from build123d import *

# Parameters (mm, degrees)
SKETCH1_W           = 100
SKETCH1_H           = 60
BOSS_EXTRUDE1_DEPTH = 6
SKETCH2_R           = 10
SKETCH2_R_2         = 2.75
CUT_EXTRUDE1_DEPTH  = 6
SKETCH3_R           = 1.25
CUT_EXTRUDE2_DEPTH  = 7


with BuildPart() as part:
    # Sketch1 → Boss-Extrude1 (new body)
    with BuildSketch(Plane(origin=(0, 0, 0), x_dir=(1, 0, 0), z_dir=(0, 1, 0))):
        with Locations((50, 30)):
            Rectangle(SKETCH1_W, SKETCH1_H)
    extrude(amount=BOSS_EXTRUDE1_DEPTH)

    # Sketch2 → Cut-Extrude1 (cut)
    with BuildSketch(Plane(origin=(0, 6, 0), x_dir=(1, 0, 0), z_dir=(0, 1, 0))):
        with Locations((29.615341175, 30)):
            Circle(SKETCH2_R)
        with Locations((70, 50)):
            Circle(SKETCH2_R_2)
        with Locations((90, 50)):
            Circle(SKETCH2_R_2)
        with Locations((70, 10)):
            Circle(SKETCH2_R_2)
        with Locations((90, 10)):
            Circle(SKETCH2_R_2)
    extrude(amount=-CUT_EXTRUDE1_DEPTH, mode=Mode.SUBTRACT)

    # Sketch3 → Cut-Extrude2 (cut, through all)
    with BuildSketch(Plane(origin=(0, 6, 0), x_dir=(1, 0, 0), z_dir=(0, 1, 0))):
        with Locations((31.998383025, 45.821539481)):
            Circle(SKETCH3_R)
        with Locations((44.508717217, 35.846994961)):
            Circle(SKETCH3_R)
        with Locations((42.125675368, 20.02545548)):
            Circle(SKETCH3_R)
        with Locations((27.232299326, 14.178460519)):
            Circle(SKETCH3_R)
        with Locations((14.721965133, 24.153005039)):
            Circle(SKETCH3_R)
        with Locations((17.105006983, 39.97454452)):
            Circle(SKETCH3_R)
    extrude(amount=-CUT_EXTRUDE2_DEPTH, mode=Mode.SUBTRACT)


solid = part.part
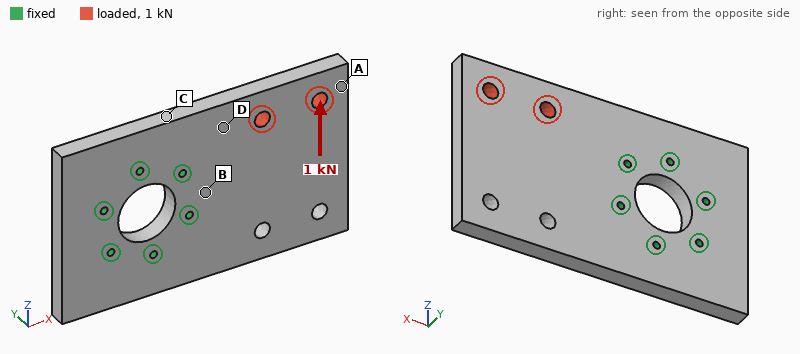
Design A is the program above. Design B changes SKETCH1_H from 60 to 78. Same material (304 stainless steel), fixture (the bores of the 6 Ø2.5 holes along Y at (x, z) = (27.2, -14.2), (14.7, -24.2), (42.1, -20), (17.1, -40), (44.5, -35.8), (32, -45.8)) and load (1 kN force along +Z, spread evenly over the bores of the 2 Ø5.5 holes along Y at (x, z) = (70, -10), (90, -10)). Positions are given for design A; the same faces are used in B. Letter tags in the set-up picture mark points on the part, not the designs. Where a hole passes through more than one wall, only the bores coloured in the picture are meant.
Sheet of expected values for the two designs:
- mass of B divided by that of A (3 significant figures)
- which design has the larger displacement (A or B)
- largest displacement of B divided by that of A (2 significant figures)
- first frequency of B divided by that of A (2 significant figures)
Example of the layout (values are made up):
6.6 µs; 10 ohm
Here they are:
1.32; A; 0.81; 0.95
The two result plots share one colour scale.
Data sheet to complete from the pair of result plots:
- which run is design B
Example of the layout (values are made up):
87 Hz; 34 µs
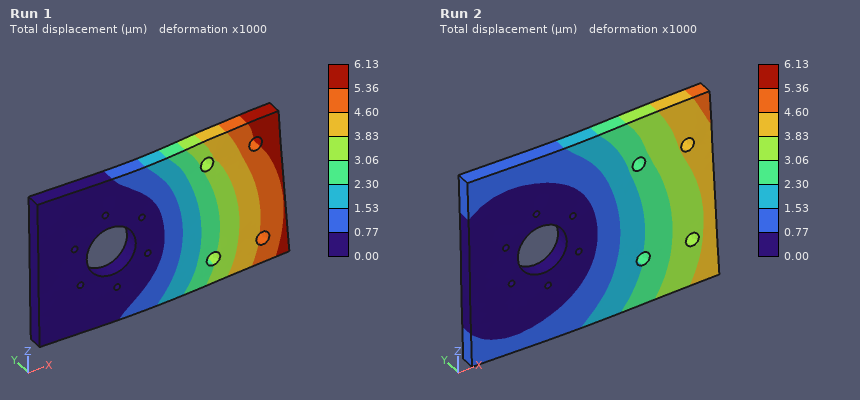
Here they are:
Run 2
